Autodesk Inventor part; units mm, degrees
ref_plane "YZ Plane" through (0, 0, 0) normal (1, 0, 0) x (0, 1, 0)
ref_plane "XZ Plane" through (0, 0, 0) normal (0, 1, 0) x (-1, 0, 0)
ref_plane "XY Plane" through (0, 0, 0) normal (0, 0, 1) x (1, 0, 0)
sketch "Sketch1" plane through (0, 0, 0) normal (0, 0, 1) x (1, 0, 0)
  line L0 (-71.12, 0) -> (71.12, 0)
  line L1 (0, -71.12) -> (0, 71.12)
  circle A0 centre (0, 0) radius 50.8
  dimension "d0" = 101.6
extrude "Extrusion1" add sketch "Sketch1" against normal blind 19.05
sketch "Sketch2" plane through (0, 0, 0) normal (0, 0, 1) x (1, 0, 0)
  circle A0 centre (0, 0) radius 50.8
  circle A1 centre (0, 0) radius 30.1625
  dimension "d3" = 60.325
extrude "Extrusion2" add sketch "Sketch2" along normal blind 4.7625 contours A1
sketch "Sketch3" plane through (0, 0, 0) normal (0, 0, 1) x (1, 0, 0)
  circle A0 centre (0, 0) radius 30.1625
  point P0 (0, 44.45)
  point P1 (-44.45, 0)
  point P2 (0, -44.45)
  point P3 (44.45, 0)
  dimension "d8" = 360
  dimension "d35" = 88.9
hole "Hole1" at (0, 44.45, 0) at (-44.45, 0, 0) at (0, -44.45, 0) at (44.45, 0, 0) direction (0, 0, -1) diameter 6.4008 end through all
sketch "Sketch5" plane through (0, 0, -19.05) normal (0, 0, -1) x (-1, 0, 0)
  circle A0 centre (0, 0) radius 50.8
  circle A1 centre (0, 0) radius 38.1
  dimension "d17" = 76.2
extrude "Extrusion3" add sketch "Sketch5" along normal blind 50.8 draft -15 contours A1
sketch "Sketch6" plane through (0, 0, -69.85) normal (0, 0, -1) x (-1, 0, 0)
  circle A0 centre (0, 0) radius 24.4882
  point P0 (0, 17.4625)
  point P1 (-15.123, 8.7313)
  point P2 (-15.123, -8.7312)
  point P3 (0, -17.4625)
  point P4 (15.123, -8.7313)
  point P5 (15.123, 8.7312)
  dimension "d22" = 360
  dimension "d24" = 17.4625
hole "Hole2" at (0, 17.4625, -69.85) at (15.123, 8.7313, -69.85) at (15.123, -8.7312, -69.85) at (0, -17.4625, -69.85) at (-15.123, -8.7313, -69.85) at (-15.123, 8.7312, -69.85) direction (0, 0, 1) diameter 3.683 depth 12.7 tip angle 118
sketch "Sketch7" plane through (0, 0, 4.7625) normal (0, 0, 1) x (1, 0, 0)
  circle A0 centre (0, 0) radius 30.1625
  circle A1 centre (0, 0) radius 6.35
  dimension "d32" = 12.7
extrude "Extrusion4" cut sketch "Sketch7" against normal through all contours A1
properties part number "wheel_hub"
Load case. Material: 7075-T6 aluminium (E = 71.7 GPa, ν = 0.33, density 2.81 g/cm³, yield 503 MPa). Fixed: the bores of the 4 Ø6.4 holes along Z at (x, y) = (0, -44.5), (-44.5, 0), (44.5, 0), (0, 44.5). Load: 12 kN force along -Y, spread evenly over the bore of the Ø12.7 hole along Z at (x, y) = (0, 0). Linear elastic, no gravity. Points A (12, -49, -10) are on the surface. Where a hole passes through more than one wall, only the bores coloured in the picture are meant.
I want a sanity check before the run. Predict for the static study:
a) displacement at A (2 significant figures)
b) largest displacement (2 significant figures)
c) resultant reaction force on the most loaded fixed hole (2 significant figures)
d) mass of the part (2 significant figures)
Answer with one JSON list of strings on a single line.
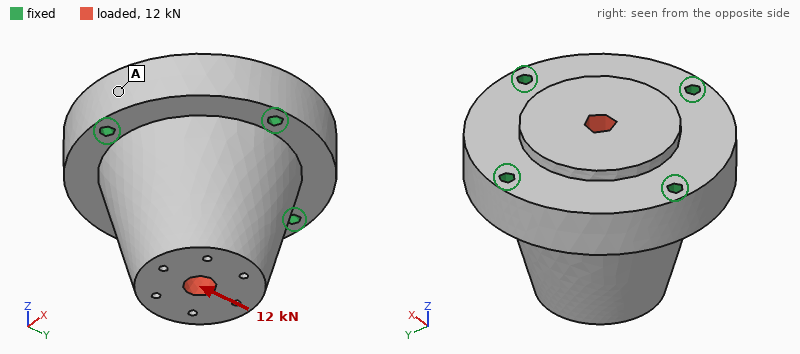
["2.1 µm", "12 µm", "5.0 kN", "880 g"]
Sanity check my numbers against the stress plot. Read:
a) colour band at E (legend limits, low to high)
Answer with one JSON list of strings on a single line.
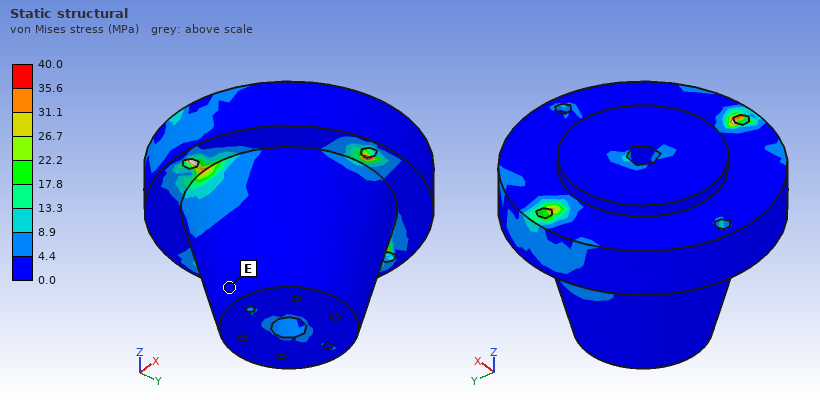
["0.0 to 4.4 MPa"]
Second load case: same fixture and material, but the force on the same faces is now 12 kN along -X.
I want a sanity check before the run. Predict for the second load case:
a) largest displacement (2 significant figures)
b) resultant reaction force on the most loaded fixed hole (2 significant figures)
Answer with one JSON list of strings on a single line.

["12 µm", "5.0 kN"]
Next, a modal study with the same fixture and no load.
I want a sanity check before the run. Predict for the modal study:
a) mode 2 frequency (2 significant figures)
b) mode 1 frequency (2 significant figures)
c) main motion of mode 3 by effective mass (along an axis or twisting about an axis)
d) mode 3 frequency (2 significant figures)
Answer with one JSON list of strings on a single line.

["8000 Hz", "8000 Hz", "along Z", "9700 Hz"]
